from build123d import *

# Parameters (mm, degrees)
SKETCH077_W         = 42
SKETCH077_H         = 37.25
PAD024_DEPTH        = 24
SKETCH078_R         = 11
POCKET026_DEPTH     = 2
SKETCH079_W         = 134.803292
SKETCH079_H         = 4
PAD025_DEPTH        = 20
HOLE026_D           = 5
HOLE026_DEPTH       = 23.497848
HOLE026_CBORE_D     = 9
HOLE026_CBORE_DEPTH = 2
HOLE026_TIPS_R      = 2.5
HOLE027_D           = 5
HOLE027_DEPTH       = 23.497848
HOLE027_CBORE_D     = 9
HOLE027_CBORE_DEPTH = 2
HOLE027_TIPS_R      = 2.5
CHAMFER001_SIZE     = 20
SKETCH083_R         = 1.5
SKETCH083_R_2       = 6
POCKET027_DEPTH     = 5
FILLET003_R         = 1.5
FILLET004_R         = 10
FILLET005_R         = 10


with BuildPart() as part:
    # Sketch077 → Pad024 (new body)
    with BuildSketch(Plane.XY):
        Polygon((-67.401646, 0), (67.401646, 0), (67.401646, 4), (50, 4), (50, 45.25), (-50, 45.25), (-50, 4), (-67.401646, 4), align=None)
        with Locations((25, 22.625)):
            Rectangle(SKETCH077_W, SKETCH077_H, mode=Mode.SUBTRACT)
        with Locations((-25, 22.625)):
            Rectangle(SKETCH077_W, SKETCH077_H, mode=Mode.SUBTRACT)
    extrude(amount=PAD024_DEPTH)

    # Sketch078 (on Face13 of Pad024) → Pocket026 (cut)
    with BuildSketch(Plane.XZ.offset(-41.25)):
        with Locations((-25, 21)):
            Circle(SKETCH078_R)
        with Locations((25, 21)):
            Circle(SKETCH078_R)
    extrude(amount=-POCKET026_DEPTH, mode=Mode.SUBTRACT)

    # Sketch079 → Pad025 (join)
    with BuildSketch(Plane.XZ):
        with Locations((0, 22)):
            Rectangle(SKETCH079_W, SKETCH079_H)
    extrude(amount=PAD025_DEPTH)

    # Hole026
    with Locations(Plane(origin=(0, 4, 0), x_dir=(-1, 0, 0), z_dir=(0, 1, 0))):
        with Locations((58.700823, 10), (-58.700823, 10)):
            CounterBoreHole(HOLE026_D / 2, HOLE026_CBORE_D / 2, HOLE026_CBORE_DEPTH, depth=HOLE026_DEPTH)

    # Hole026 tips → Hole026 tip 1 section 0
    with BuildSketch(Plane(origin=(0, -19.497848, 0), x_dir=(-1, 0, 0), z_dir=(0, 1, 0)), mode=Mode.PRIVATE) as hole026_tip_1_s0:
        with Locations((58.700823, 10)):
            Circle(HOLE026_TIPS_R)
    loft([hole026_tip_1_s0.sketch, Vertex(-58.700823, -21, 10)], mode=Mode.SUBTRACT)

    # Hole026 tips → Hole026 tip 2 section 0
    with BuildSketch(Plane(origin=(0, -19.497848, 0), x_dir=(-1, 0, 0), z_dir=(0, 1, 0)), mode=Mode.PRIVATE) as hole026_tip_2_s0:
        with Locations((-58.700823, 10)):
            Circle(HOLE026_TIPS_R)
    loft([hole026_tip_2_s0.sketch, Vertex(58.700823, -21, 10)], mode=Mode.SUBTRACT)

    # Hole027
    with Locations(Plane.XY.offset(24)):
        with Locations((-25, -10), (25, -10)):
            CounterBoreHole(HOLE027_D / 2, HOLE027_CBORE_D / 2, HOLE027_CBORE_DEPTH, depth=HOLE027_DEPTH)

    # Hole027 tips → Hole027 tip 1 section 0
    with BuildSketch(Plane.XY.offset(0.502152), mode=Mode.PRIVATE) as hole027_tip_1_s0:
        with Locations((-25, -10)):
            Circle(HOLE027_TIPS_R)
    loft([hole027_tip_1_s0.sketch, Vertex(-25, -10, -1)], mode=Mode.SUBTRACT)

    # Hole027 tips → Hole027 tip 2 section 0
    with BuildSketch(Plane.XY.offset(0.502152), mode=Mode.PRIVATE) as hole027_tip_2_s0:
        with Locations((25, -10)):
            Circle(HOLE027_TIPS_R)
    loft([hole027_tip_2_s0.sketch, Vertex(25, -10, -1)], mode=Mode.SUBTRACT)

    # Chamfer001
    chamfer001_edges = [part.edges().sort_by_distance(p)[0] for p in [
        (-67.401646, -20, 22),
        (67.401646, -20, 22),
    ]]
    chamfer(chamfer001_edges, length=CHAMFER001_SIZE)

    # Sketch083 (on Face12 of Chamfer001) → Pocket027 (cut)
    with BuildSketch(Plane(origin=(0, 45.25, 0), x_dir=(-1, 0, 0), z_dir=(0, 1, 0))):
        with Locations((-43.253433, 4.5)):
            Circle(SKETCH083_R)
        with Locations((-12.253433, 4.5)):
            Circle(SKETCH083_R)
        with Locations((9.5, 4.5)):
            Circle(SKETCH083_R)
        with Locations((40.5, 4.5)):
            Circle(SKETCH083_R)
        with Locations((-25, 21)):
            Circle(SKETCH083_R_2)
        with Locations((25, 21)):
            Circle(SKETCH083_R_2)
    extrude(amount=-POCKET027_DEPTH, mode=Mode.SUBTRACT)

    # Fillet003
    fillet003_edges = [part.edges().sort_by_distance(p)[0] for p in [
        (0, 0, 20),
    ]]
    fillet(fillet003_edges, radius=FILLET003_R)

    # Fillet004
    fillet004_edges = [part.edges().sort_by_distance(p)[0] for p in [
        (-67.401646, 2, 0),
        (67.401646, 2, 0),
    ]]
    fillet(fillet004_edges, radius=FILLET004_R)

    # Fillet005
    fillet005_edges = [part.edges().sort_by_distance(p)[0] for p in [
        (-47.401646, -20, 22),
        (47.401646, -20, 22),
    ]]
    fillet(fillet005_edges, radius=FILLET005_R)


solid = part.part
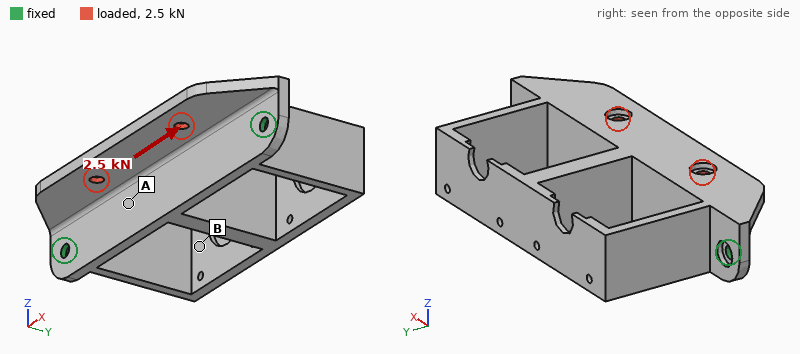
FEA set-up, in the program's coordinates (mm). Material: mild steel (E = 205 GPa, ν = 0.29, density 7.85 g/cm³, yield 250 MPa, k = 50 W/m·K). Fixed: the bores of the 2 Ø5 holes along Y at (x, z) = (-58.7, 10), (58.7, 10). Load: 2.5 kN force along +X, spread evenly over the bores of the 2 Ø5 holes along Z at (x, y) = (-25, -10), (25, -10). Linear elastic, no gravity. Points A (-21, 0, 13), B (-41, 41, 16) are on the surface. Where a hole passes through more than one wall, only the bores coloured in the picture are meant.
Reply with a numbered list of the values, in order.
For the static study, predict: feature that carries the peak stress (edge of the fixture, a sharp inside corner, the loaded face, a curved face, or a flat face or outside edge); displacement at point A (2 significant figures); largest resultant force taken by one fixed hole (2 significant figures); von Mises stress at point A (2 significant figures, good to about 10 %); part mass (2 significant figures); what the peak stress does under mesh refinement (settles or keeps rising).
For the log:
1. edge of the fixture
2. 3.1 µm
3. 1.3 kN
4. 11 MPa
5. 340 g
6. keeps rising
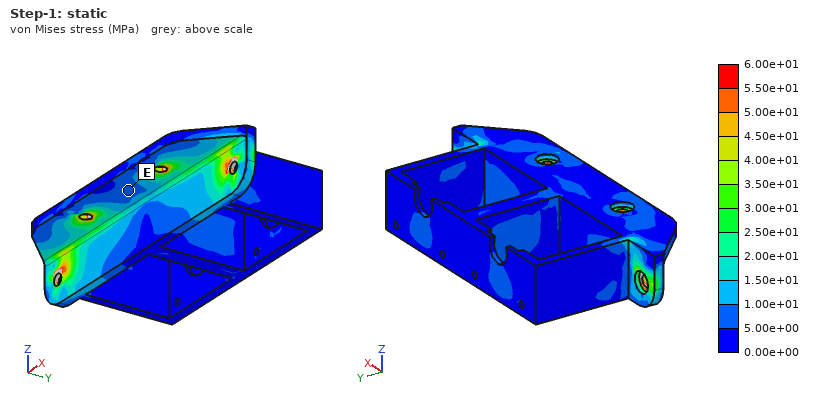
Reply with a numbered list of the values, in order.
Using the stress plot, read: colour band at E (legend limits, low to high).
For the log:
1. 5.00e+00 to 1.00e+01 MPa
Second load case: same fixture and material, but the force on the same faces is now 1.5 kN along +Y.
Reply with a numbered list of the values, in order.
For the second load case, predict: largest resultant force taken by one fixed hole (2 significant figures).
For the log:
1. 780 N
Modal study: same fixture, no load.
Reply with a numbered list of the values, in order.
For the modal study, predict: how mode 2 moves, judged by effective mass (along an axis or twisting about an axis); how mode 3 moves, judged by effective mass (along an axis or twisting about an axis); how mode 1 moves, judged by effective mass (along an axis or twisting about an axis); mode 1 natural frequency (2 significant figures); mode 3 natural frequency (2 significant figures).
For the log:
1. along X
2. along Y
3. along Z
4. 800 Hz
5. 2300 Hz
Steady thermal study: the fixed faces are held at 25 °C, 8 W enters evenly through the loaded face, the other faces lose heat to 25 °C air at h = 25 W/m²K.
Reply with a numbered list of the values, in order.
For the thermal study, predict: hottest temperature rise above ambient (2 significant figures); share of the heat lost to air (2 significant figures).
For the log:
1. 21 K
2. 54 %
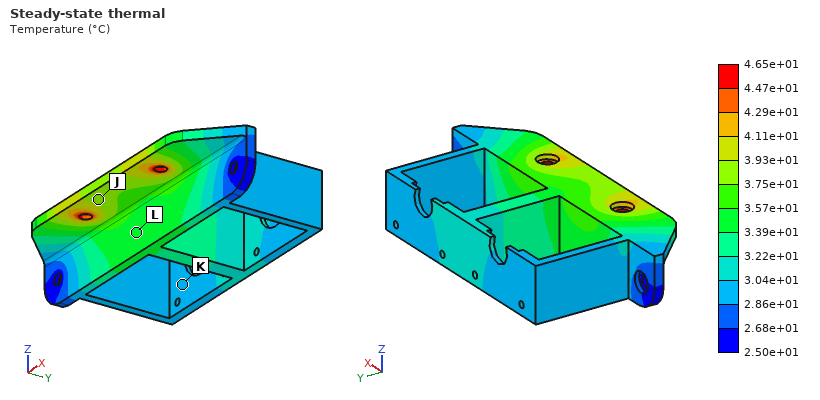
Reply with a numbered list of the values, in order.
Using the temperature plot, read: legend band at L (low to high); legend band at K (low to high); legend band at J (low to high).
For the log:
1. 3.39e+01 to 3.57e+01 °C
2. 2.86e+01 to 3.04e+01 °C
3. 3.75e+01 to 3.93e+01 °C
